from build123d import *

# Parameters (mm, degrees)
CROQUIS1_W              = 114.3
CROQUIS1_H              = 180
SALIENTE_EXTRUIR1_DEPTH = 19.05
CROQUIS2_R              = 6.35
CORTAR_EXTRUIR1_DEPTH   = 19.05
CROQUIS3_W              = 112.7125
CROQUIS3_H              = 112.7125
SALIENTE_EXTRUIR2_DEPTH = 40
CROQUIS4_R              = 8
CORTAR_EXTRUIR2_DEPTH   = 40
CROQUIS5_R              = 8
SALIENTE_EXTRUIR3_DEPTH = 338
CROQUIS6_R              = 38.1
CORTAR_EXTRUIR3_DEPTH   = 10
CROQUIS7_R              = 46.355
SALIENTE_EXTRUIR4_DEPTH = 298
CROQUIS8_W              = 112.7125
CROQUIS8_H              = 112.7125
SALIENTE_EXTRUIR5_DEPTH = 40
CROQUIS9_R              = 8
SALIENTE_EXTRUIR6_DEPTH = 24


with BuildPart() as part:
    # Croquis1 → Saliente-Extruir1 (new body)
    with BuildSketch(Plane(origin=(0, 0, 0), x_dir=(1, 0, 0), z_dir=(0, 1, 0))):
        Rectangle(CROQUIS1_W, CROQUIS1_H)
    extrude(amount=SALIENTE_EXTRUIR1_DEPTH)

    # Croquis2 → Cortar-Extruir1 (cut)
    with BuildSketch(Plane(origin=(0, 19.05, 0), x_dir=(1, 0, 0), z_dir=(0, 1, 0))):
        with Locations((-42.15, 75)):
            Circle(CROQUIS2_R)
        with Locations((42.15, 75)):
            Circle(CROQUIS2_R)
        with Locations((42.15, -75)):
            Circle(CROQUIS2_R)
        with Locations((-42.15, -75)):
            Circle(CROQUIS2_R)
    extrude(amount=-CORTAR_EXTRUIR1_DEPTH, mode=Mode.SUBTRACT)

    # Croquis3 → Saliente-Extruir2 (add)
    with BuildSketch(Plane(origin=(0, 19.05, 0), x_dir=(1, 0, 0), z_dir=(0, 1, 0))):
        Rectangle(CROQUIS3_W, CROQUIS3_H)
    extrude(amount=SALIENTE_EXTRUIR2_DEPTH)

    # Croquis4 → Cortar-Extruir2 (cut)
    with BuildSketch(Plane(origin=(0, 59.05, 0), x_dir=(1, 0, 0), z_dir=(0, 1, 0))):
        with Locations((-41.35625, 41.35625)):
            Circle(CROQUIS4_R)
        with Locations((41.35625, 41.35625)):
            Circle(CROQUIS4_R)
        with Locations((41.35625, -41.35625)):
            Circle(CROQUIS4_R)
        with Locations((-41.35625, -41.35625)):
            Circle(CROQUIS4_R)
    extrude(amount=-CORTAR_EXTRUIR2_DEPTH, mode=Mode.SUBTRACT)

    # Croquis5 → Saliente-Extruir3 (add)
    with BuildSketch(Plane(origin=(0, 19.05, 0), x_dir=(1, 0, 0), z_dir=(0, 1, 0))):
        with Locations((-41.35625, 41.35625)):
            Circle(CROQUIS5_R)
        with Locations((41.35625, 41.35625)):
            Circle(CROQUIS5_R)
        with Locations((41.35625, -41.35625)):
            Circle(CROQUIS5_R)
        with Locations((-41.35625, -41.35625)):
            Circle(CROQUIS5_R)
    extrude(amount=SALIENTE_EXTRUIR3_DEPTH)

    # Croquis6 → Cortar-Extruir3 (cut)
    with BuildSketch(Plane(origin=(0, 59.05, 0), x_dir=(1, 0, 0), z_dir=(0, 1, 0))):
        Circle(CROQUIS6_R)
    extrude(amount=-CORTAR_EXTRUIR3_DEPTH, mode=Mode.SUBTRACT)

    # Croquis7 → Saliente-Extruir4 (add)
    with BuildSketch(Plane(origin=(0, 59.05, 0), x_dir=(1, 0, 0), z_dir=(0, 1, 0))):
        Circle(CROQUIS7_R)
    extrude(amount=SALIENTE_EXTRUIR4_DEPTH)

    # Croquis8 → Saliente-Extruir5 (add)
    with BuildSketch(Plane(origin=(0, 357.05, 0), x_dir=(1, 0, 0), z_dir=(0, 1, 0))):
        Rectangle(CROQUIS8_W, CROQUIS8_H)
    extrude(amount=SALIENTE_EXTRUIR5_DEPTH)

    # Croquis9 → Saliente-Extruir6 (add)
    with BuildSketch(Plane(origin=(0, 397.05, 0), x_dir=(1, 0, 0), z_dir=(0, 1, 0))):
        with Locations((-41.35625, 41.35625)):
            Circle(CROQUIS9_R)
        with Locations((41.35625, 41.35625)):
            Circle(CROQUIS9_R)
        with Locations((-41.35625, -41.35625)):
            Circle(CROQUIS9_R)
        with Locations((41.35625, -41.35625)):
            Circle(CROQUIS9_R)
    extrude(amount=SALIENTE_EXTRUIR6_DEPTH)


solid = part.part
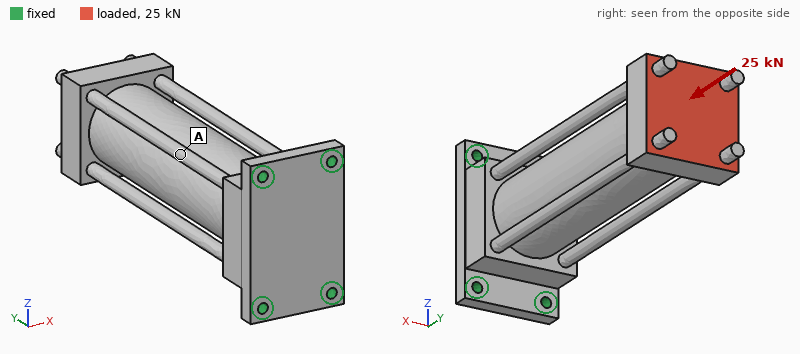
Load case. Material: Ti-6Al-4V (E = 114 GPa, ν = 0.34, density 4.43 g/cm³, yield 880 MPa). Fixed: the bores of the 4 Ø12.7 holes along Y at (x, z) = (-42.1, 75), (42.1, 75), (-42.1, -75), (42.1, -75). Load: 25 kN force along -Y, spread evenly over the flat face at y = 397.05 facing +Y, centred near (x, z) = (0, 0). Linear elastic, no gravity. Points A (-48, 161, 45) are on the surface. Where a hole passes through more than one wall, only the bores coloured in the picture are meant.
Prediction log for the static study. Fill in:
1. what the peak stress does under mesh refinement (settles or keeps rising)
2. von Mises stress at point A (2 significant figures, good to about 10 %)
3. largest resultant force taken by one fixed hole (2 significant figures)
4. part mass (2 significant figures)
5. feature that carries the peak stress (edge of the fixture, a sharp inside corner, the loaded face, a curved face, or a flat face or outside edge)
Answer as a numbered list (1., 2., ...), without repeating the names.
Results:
1. keeps rising
2. 4.3 MPa
3. 6.9 kN
4. 16 kg
5. edge of the fixture
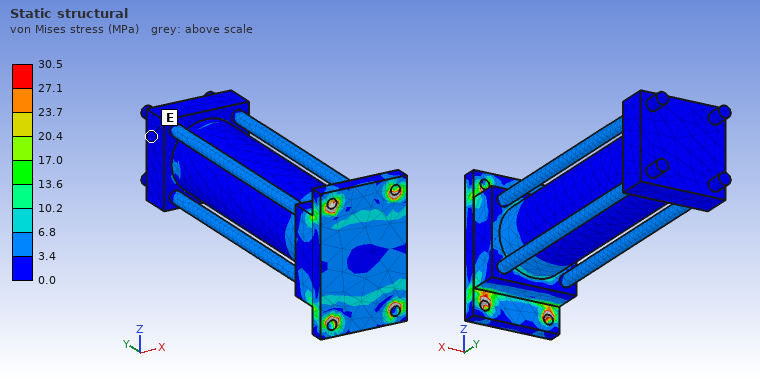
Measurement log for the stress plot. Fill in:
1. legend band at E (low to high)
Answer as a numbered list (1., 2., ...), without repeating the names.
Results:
1. 0.0 to 3.4 MPa
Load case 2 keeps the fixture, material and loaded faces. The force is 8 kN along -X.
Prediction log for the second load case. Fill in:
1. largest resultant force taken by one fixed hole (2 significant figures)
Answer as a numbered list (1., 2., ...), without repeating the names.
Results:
1. 20 kN
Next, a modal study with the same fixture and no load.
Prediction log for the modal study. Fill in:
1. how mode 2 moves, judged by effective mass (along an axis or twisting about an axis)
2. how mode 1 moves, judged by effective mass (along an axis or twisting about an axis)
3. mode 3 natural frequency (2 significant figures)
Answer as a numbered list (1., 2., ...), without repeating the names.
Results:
1. along Z
2. along X
3. 760 Hz
